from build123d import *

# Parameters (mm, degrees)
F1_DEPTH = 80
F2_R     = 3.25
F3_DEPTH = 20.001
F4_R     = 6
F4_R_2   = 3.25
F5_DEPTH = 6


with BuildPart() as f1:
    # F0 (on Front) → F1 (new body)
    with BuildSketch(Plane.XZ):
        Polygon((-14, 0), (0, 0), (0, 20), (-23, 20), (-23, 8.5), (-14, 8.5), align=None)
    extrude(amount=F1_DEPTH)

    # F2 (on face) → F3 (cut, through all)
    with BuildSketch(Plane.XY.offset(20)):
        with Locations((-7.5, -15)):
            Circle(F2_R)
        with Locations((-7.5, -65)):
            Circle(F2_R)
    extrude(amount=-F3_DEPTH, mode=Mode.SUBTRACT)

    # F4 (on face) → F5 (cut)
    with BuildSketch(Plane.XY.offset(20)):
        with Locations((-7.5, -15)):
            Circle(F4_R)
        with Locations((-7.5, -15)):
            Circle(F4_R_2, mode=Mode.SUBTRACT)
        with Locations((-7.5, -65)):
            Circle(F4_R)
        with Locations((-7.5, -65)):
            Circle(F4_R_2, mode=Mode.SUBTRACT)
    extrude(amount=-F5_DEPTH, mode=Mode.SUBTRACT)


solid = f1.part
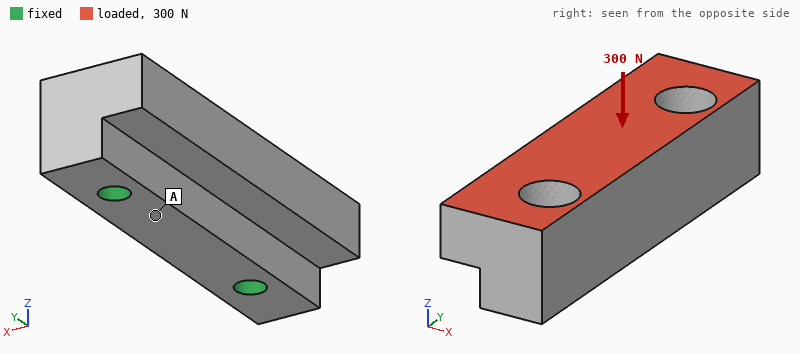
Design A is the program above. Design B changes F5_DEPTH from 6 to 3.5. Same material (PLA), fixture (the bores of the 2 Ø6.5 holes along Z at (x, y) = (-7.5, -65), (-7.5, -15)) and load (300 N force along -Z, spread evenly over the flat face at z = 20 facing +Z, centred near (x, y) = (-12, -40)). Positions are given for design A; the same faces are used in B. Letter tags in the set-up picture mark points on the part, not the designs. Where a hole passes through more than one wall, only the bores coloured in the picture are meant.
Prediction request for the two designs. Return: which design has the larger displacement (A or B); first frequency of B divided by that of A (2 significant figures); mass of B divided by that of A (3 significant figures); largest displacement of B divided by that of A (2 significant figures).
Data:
A
1.2
1.01
0.80
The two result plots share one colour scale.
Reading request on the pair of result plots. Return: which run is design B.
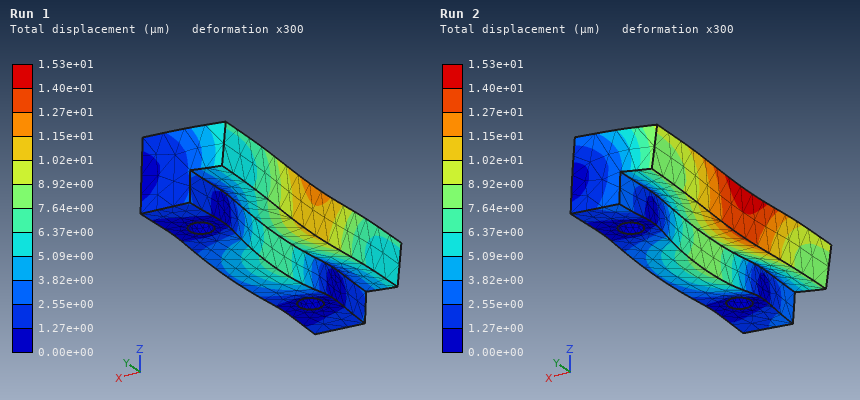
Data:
Run 1
